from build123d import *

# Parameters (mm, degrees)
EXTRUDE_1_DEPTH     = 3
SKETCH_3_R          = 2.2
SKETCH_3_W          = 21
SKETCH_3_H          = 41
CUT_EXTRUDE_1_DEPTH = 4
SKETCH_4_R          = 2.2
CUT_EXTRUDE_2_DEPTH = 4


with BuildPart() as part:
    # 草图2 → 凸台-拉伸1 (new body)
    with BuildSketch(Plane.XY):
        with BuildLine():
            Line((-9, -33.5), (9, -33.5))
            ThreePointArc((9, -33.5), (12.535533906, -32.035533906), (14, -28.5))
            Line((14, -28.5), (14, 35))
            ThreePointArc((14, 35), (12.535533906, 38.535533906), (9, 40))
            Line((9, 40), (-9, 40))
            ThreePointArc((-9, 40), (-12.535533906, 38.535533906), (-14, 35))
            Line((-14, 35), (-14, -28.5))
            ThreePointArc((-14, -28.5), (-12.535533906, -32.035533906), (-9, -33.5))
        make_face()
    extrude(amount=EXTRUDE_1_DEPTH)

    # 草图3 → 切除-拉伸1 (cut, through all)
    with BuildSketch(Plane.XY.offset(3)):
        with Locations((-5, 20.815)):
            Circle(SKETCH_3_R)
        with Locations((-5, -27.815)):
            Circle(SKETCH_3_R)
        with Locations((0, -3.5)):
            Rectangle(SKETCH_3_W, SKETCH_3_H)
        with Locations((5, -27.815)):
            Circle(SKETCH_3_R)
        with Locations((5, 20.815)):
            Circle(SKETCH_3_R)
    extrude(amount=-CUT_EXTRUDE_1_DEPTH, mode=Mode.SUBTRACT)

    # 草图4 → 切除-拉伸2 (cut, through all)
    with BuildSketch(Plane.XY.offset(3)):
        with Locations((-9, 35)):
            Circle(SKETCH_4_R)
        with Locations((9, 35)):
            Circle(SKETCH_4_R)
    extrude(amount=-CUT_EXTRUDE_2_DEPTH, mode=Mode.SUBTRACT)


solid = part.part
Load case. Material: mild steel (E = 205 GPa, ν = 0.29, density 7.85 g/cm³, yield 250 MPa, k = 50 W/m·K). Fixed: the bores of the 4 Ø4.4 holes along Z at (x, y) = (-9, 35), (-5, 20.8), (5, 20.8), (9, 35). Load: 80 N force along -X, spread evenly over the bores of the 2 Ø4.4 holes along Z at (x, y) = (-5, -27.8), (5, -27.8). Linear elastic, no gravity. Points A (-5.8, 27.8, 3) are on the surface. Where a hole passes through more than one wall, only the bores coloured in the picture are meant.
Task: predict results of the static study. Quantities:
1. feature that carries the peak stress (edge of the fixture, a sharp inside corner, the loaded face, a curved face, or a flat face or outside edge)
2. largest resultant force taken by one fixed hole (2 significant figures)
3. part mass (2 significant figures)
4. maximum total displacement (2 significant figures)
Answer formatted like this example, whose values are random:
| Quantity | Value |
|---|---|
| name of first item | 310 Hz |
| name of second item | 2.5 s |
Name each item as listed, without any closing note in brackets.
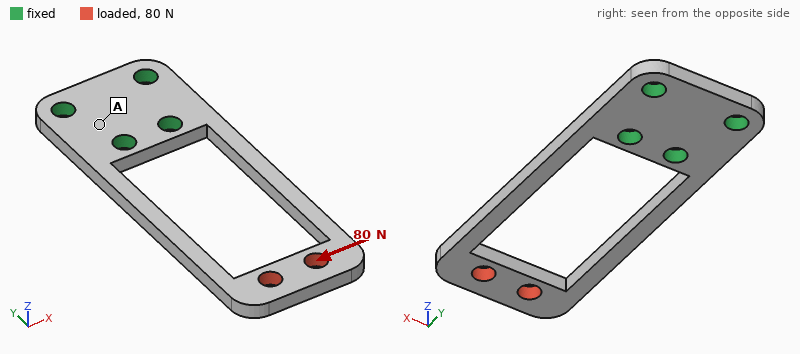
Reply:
| Quantity | Value |
|---|---|
| feature that carries the peak stress | a flat face or outside edge |
| largest resultant force taken by one fixed hole | 120 N |
| part mass | 26 g |
| maximum total displacement | 0.15 mm |
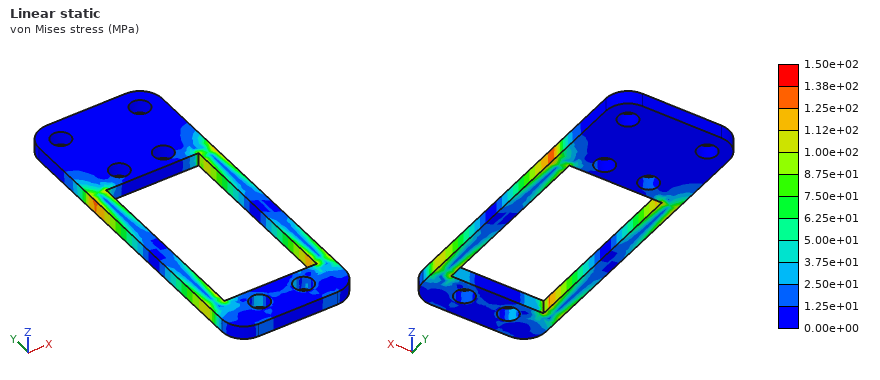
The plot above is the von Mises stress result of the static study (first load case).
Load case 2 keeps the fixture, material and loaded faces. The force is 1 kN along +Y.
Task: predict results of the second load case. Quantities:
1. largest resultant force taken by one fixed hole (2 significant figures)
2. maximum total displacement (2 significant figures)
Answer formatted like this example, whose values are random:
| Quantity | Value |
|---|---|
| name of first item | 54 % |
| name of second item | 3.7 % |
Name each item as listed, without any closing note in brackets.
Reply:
| Quantity | Value |
|---|---|
| largest resultant force taken by one fixed hole | 280 N |
| maximum total displacement | 21 µm |
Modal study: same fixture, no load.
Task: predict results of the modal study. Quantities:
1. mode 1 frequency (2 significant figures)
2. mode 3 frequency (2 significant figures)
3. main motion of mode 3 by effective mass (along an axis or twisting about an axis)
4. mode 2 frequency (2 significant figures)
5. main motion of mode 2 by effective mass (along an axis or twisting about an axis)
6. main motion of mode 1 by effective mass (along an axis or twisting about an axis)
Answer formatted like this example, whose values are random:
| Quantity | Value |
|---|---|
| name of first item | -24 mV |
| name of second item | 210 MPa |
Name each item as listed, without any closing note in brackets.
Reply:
| Quantity | Value |
|---|---|
| mode 1 frequency | 560 Hz |
| mode 3 frequency | 1800 Hz |
| main motion of mode 3 by effective mass | twisting about Y |
| mode 2 frequency | 1300 Hz |
| main motion of mode 2 by effective mass | along X |
| main motion of mode 1 by effective mass | along Z |
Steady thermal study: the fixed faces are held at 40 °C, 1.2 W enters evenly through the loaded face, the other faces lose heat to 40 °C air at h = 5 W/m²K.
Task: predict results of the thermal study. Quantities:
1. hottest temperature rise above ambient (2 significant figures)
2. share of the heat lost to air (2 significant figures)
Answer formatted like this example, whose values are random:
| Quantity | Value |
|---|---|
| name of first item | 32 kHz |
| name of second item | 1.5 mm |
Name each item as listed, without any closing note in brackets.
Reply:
| Quantity | Value |
|---|---|
| hottest temperature rise above ambient | 48 K |
| share of the heat lost to air | 22 % |
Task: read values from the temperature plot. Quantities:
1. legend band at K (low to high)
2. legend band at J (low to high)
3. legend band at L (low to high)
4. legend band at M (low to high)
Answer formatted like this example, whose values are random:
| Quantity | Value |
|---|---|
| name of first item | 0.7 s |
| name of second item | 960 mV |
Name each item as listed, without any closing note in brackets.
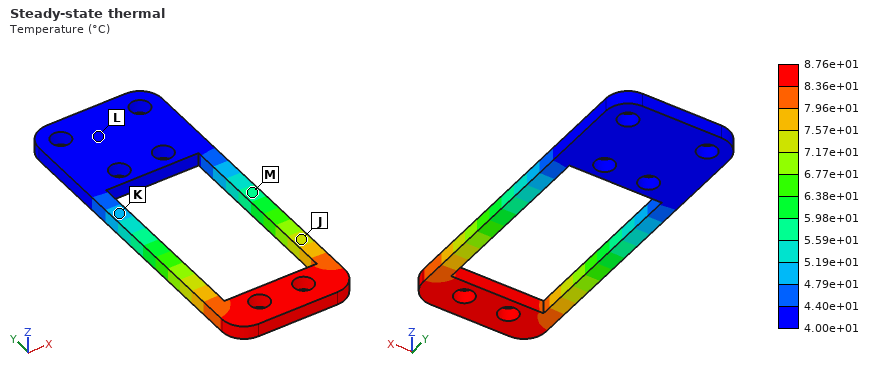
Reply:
| Quantity | Value |
|---|---|
| legend band at K | 4.79e+01 to 5.19e+01 °C |
| legend band at J | 7.17e+01 to 7.57e+01 °C |
| legend band at L | 4.00e+01 to 4.40e+01 °C |
| legend band at M | 5.59e+01 to 5.98e+01 °C |
